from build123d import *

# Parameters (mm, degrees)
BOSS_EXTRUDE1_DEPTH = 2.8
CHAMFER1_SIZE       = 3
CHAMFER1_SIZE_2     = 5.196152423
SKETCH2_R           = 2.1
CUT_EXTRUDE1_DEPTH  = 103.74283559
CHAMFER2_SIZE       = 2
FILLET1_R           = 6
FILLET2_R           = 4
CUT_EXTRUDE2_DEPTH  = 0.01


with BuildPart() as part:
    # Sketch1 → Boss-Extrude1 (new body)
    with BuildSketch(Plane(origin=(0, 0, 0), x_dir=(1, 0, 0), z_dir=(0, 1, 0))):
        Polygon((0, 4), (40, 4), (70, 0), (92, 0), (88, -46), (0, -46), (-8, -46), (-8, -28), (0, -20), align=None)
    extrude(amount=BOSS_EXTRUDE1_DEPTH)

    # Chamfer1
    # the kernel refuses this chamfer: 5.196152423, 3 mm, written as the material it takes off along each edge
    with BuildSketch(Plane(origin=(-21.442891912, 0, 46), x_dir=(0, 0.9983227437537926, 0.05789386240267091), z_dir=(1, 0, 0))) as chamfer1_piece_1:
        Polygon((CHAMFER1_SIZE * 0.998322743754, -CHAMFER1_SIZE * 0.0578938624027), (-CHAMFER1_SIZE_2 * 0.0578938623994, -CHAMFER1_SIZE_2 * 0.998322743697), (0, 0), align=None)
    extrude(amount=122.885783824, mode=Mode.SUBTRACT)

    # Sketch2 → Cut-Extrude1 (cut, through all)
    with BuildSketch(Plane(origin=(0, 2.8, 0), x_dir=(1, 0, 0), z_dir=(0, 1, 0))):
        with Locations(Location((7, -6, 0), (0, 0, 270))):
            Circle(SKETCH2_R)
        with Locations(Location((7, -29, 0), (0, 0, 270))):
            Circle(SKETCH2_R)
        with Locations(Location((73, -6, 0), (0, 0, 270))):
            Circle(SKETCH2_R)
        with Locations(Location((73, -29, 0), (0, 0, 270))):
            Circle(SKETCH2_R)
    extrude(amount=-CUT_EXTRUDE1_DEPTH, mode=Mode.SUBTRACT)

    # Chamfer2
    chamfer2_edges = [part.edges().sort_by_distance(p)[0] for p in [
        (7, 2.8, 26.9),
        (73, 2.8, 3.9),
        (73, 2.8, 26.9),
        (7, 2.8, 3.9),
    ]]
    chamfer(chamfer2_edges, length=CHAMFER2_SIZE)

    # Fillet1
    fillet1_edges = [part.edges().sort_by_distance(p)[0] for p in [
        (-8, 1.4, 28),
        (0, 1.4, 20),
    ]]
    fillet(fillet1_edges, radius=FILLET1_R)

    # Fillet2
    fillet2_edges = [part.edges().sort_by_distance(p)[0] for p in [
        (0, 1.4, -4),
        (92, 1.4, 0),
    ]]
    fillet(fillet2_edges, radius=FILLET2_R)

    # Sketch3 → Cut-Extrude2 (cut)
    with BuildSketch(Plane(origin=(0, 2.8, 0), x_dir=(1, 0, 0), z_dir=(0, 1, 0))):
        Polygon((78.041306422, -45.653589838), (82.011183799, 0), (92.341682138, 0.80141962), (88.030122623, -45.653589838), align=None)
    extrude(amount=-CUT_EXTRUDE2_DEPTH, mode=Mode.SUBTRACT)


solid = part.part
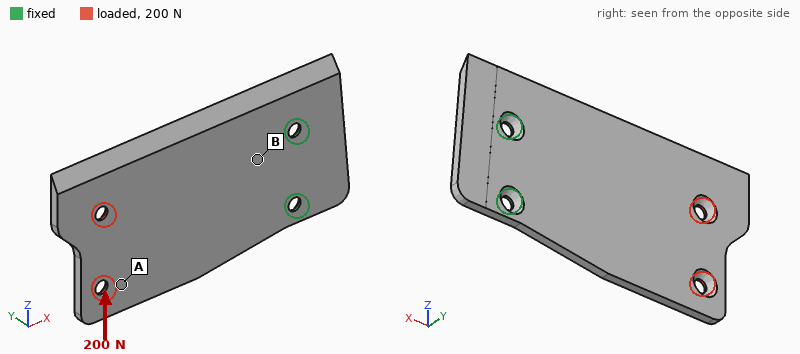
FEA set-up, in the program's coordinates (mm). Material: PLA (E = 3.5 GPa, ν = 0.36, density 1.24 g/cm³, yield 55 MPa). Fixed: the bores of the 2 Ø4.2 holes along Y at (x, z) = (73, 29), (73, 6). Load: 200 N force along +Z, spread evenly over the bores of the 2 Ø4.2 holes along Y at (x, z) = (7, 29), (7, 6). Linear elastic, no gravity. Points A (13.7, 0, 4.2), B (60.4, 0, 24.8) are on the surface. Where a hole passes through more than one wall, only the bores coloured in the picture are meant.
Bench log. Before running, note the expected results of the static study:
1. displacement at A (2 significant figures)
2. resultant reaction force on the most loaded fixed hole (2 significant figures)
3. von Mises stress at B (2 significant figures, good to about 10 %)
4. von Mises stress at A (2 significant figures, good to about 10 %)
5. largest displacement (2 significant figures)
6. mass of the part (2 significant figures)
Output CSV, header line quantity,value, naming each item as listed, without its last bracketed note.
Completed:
quantity,value
displacement at A,0.85 mm
resultant reaction force on the most loaded fixed hole,550 N
von Mises stress at B,12 MPa
von Mises stress at A,5.3 MPa
largest displacement,1.3 mm
mass of the part,14 g
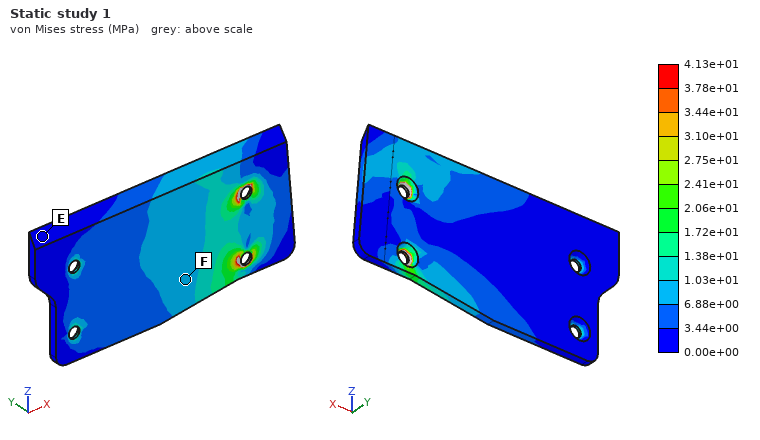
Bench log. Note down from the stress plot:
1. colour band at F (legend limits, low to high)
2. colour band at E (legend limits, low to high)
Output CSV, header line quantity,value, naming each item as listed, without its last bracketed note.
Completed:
quantity,value
colour band at F,6.88e+00 to 1.03e+01 MPa
colour band at E,0.00e+00 to 3.44e+00 MPa
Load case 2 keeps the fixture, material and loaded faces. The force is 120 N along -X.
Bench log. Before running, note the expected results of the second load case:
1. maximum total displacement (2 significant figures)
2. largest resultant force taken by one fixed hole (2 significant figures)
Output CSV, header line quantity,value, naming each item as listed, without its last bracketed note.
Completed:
quantity,value
maximum total displacement,1.2 mm
largest resultant force taken by one fixed hole,61 N
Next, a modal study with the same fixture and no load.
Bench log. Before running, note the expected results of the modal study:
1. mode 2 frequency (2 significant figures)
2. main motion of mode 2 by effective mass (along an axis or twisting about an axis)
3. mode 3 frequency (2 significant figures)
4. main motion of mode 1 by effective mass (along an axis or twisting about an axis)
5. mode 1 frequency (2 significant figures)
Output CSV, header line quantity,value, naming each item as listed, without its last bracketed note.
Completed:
quantity,value
mode 2 frequency,420 Hz
main motion of mode 2 by effective mass,twisting about X
mode 3 frequency,710 Hz
main motion of mode 1 by effective mass,along Y
mode 1 frequency,110 Hz
